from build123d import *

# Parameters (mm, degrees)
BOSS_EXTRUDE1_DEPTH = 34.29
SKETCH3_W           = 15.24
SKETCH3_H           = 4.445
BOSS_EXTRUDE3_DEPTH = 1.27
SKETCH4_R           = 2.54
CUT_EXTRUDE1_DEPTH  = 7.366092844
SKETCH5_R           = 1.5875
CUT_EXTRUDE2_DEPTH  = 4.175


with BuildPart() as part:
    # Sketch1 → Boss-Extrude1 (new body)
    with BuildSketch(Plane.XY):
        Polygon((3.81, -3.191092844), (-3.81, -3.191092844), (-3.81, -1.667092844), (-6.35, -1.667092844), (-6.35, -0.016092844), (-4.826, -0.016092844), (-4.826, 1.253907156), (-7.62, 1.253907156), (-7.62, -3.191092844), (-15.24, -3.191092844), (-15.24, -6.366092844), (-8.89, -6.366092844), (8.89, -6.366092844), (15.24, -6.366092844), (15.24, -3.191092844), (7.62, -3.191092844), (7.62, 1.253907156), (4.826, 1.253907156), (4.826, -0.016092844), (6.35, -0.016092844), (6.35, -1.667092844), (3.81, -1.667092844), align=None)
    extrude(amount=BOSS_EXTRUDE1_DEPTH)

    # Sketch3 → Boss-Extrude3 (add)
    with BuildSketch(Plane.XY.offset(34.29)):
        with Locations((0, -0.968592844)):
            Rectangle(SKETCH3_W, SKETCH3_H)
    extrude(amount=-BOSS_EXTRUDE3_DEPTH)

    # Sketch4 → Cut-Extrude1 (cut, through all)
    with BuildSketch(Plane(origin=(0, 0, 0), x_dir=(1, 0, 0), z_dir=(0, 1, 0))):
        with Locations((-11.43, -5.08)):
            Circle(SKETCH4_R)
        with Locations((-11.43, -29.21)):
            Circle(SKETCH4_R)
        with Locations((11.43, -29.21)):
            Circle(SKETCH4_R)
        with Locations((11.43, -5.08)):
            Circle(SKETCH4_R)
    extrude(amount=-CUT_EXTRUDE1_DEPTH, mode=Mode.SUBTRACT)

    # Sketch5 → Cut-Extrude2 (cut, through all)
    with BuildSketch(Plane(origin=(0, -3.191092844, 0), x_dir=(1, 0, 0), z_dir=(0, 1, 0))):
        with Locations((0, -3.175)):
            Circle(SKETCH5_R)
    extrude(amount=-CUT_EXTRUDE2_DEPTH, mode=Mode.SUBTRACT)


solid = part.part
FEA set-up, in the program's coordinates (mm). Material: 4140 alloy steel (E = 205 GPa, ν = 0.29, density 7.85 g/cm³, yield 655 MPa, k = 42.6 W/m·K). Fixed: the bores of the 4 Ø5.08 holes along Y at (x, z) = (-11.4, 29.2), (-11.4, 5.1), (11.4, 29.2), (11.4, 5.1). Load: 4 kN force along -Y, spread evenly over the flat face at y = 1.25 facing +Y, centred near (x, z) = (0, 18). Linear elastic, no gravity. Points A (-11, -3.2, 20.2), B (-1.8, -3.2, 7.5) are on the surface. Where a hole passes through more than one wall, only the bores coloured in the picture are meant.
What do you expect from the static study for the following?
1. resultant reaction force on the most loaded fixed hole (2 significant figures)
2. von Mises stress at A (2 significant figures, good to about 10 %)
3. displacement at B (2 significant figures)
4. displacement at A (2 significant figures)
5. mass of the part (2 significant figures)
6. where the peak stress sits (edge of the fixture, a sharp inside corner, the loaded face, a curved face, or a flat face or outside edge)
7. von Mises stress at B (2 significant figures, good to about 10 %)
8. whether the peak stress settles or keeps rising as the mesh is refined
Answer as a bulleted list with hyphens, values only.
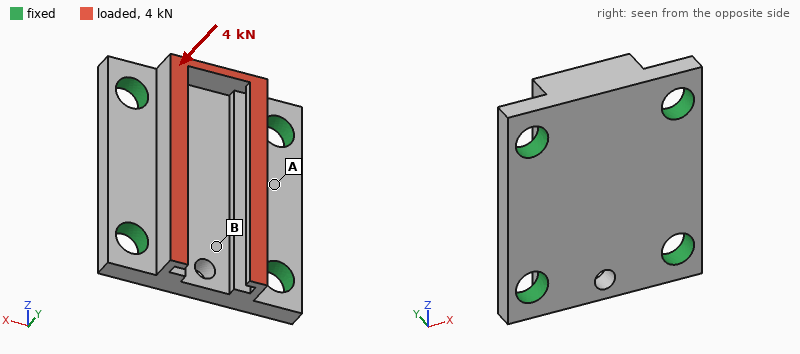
- 1.1 kN
- 18 MPa
- 5.2 µm
- 2.6 µm
- 30 g
- edge of the fixture
- 42 MPa
- keeps rising
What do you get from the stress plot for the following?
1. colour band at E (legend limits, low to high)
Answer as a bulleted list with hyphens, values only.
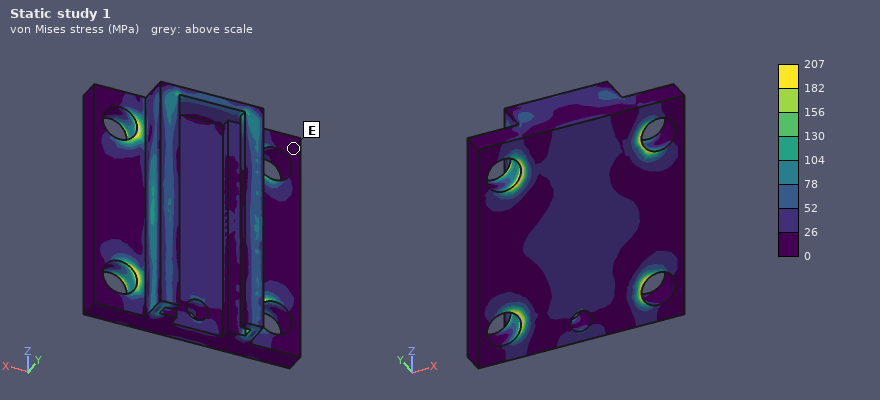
- 0 to 26 MPa
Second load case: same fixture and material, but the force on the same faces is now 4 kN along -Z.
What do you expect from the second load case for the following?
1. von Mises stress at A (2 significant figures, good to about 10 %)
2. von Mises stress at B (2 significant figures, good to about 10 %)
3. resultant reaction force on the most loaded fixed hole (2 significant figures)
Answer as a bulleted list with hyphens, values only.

- 18 MPa
- 16 MPa
- 1.1 kN
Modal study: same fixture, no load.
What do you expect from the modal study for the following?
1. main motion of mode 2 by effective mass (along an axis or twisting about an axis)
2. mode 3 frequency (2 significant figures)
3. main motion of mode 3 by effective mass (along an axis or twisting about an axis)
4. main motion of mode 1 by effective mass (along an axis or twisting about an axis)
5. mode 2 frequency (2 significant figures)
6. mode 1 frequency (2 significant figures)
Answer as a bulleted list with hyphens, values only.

- twisting about X
- 39 kHz
- twisting about Z
- along Y
- 35 kHz
- 25 kHz
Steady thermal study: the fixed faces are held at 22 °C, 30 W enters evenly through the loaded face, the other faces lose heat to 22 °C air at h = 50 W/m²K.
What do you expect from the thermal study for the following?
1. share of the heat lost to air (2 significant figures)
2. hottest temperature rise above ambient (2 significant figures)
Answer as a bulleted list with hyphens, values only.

- 8.2 %
- 48 K
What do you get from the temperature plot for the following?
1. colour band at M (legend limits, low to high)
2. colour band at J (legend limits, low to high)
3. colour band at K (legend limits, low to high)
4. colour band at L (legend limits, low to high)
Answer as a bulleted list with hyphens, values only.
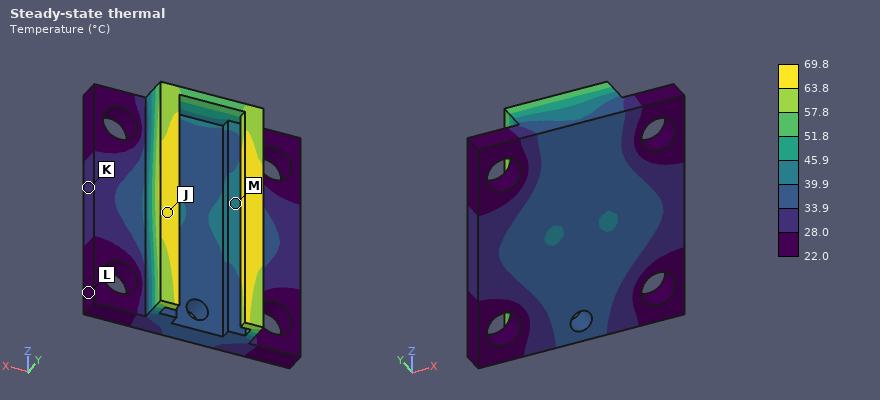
- 39.9 to 45.9 °C
- 63.8 to 69.8 °C
- 28.0 to 33.9 °C
- 22.0 to 28.0 °C
